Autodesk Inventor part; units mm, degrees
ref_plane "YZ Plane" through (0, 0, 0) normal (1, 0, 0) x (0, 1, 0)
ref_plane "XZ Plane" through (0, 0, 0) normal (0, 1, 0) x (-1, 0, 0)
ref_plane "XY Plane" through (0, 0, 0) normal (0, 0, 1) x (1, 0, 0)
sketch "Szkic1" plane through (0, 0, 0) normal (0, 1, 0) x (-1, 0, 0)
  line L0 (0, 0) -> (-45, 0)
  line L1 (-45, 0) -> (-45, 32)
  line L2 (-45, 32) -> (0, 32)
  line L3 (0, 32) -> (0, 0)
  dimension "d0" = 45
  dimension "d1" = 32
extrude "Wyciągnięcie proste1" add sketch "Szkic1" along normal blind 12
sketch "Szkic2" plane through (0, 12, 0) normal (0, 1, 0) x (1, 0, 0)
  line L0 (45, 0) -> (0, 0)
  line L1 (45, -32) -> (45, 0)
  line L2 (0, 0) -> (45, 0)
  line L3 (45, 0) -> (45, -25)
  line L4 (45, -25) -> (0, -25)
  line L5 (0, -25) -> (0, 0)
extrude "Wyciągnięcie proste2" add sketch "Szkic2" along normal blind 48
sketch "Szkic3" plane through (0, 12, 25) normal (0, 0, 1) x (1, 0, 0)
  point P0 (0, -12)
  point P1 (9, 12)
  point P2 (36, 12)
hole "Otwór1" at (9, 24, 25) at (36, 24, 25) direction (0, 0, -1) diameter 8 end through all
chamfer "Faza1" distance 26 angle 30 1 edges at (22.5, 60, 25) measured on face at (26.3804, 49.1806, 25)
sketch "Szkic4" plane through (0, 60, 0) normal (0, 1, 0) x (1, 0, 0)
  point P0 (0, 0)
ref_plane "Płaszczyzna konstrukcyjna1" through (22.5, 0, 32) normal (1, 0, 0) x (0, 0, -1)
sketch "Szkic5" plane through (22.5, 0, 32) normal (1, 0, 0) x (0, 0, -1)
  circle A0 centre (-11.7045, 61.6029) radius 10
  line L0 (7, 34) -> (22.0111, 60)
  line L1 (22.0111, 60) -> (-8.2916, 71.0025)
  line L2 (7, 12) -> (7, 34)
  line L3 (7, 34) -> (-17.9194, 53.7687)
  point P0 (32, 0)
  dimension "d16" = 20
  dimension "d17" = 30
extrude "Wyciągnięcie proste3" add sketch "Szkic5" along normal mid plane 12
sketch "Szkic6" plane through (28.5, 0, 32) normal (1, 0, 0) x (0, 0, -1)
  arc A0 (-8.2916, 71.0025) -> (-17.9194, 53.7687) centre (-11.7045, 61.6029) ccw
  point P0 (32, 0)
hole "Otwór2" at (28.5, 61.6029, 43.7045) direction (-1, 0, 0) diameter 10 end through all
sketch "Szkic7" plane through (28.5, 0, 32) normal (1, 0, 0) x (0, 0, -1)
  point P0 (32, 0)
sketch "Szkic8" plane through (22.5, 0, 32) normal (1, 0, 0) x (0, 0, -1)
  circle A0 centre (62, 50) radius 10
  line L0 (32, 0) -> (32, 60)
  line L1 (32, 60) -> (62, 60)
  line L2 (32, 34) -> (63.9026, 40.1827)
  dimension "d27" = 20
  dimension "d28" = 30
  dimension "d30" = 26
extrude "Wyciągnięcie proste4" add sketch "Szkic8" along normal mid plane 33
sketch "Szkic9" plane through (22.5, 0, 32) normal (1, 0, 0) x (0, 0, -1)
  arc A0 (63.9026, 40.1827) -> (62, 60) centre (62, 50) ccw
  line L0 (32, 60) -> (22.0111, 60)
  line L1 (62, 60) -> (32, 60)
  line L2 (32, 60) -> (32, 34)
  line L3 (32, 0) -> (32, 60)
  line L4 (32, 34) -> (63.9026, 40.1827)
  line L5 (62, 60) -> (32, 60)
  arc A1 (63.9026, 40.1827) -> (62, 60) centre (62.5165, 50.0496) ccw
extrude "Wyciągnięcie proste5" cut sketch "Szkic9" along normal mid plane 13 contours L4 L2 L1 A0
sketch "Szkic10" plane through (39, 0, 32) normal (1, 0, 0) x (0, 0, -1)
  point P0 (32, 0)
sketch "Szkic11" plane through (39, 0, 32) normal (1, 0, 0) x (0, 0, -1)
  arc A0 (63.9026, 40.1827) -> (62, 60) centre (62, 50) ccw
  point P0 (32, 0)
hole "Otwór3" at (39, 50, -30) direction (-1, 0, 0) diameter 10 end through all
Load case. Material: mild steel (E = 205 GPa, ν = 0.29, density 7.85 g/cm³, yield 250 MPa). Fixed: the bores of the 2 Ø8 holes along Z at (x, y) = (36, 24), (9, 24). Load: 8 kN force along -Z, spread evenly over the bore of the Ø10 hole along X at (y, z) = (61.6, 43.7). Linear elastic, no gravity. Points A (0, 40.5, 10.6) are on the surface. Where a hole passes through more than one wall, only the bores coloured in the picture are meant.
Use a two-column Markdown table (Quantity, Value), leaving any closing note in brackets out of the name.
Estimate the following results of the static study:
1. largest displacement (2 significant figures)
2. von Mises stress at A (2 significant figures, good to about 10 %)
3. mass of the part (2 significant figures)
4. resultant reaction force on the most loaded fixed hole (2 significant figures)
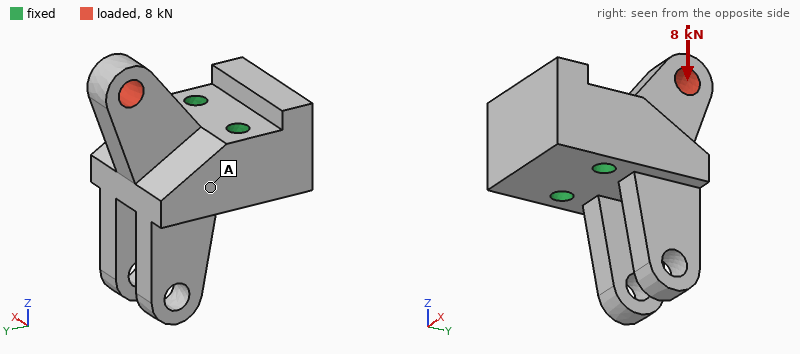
| Quantity | Value |
|---|---|
| largest displacement | 51 µm |
| von Mises stress at A | 13 MPa |
| mass of the part | 670 g |
| resultant reaction force on the most loaded fixed hole | 4.0 kN |
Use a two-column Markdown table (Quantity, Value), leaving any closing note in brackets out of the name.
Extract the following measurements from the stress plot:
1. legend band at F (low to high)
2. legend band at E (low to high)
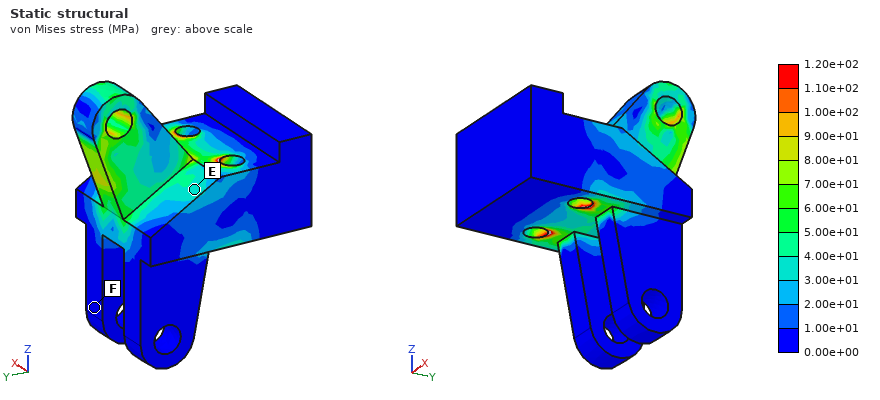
| Quantity | Value |
|---|---|
| legend band at F | 0.00e+00 to 1.00e+01 MPa |
| legend band at E | 3.00e+01 to 4.00e+01 MPa |
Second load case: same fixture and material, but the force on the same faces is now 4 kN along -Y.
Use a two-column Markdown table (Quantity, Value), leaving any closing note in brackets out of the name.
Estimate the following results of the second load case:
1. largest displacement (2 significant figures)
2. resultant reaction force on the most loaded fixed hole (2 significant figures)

| Quantity | Value |
|---|---|
| largest displacement | 34 µm |
| resultant reaction force on the most loaded fixed hole | 2.2 kN |
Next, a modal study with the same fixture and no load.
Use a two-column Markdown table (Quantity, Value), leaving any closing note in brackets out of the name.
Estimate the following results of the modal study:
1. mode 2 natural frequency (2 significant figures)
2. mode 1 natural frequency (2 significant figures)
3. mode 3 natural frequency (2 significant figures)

| Quantity | Value |
|---|---|
| mode 2 natural frequency | 5400 Hz |
| mode 1 natural frequency | 5200 Hz |
| mode 3 natural frequency | 6200 Hz |
